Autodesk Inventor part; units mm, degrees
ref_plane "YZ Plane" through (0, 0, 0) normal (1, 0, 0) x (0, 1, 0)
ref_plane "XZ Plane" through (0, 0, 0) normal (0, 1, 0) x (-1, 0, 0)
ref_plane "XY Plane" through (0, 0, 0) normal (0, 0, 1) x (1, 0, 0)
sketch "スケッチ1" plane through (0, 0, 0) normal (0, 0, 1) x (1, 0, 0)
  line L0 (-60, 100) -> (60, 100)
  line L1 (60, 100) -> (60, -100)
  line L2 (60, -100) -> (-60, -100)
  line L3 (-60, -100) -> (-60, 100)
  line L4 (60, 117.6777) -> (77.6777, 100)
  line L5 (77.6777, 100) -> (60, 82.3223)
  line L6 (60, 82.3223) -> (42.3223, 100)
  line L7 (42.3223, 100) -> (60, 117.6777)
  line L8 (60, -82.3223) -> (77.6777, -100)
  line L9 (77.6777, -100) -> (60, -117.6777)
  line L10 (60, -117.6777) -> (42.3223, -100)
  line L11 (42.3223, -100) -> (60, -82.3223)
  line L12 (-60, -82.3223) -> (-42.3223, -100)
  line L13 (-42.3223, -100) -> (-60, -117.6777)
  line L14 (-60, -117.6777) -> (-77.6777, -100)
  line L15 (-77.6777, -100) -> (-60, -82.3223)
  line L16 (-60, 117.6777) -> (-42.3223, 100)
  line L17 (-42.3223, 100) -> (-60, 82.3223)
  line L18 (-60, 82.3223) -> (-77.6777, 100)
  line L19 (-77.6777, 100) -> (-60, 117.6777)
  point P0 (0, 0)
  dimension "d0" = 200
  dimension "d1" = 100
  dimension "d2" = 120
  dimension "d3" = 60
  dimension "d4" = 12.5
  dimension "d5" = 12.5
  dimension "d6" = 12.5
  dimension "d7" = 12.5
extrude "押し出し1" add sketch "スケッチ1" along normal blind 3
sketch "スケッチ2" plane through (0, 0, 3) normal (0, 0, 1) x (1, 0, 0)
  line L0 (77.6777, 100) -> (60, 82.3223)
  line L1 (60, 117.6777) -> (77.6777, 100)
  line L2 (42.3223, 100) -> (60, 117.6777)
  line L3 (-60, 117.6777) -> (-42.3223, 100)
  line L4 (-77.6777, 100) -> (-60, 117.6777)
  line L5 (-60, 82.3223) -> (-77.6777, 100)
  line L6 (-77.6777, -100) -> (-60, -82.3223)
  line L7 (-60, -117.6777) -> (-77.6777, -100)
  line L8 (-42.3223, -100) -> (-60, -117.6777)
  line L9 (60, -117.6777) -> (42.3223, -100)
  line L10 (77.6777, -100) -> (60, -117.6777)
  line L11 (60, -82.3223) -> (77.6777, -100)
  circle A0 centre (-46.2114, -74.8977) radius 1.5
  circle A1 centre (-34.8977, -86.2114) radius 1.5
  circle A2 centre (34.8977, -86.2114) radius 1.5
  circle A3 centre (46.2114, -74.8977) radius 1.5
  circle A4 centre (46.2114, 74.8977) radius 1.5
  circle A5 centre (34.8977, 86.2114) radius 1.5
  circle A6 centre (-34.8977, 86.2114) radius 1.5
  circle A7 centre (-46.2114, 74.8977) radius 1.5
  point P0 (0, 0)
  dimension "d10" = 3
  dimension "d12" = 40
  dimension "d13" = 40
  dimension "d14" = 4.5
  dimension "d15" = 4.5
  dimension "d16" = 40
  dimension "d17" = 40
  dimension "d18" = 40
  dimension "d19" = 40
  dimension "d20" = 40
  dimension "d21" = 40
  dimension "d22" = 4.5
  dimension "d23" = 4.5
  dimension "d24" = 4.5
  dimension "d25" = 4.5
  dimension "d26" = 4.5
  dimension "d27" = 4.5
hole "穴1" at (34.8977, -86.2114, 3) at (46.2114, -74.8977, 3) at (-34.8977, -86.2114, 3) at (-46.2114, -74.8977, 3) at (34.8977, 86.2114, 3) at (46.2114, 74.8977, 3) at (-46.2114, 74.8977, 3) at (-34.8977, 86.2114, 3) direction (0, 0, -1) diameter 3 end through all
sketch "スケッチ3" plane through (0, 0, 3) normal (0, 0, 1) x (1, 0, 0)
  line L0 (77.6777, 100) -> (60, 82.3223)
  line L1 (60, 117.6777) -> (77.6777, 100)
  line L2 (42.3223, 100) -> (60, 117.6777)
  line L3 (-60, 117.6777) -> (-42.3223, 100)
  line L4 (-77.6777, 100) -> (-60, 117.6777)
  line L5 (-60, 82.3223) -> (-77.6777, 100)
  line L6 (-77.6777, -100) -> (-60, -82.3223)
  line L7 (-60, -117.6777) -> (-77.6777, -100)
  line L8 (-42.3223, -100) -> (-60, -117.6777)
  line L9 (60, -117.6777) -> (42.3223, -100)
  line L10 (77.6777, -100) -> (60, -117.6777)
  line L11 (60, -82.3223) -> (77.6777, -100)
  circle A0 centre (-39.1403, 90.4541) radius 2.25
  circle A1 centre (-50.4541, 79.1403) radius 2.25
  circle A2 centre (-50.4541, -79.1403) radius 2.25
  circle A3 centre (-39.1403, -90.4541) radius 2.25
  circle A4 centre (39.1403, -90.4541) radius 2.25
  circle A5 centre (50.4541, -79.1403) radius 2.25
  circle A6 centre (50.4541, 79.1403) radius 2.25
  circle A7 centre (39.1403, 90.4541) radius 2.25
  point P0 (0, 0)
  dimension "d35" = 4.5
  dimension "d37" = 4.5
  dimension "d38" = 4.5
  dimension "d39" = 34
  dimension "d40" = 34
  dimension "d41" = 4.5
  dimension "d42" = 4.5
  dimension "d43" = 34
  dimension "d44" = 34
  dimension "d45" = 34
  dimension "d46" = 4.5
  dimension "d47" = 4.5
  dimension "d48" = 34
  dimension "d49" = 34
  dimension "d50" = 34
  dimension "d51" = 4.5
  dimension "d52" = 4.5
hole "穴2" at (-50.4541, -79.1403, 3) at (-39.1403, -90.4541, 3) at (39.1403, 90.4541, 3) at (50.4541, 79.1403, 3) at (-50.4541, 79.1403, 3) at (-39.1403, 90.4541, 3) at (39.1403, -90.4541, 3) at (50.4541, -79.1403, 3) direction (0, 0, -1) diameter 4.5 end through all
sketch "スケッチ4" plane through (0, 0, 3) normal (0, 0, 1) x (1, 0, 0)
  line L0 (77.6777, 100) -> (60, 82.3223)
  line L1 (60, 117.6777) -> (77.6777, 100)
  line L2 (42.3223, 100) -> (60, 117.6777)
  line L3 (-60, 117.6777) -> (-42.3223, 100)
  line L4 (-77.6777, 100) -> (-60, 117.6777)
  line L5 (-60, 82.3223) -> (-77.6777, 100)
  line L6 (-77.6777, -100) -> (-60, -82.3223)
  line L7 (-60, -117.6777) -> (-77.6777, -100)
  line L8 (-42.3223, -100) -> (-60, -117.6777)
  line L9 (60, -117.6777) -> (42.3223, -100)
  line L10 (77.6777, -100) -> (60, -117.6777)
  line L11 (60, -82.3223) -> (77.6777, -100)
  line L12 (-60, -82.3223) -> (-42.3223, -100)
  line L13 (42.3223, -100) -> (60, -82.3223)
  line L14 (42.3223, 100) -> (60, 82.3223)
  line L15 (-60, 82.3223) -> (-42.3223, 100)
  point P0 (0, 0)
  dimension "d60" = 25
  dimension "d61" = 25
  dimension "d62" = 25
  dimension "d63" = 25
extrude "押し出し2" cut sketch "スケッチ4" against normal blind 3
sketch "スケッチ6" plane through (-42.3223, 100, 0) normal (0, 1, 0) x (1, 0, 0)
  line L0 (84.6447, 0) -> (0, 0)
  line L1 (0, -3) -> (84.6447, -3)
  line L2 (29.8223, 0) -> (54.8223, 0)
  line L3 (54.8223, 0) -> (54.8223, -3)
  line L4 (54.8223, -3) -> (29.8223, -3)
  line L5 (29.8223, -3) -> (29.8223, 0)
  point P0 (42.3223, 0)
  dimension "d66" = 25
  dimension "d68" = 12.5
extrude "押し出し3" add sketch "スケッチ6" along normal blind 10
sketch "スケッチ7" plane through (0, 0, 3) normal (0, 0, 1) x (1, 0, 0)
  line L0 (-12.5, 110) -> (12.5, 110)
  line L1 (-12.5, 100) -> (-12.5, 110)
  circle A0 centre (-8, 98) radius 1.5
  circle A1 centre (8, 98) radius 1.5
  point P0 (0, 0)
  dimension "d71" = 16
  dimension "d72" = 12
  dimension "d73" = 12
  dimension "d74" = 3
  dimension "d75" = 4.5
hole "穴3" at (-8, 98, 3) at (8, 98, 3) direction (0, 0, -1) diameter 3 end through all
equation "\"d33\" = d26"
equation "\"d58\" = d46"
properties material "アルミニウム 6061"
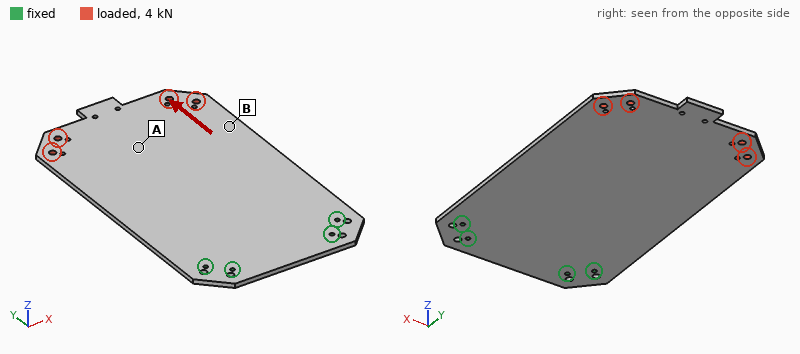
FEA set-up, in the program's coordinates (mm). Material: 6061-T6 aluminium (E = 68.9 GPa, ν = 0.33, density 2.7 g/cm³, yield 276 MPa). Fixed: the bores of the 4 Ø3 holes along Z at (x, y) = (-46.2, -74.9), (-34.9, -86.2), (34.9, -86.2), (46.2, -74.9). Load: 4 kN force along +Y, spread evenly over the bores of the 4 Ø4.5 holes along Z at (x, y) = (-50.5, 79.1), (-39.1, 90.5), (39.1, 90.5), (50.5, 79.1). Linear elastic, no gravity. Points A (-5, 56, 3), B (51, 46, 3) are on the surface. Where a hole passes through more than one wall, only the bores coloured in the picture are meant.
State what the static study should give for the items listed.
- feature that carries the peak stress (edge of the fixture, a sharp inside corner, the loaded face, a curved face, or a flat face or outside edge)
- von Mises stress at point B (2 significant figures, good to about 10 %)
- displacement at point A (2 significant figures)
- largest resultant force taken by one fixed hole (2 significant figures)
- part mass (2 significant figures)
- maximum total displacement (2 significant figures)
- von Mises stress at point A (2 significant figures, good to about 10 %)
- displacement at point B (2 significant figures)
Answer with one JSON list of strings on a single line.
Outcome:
["the loaded face", "15 MPa", "23 µm", "1.1 kN", "190 g", "37 µm", "5.3 MPa", "25 µm"]
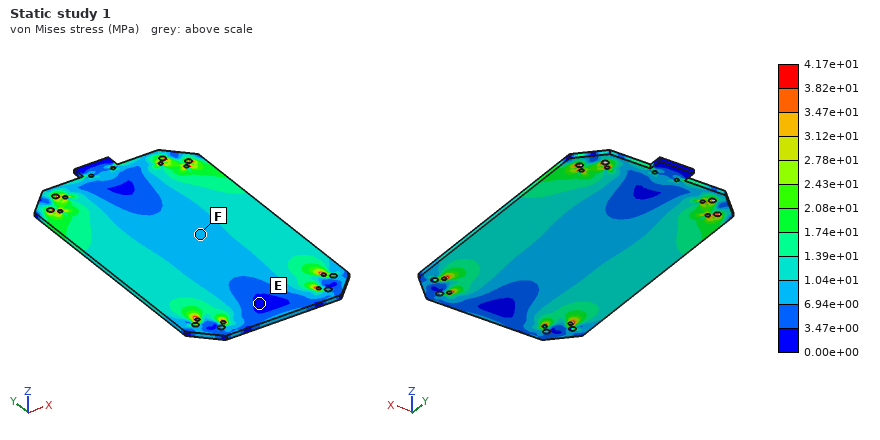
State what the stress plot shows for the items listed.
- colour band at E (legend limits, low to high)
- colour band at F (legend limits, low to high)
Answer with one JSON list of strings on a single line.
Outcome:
["0.00e+00 to 3.47e+00 MPa", "6.94e+00 to 1.04e+01 MPa"]
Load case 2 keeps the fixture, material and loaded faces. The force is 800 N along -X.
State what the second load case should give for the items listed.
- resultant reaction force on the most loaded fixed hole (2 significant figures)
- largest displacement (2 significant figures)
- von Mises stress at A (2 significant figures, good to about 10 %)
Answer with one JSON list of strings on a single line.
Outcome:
["1.1 kN", "72 µm", "5.6 MPa"]
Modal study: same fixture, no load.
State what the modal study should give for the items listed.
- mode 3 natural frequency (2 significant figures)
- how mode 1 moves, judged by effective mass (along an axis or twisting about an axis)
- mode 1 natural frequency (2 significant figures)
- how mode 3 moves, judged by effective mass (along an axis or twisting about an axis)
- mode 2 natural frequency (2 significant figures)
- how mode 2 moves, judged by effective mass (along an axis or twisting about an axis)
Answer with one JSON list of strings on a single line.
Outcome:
["470 Hz", "along Z", "76 Hz", "along Z", "280 Hz", "twisting about Y"]
